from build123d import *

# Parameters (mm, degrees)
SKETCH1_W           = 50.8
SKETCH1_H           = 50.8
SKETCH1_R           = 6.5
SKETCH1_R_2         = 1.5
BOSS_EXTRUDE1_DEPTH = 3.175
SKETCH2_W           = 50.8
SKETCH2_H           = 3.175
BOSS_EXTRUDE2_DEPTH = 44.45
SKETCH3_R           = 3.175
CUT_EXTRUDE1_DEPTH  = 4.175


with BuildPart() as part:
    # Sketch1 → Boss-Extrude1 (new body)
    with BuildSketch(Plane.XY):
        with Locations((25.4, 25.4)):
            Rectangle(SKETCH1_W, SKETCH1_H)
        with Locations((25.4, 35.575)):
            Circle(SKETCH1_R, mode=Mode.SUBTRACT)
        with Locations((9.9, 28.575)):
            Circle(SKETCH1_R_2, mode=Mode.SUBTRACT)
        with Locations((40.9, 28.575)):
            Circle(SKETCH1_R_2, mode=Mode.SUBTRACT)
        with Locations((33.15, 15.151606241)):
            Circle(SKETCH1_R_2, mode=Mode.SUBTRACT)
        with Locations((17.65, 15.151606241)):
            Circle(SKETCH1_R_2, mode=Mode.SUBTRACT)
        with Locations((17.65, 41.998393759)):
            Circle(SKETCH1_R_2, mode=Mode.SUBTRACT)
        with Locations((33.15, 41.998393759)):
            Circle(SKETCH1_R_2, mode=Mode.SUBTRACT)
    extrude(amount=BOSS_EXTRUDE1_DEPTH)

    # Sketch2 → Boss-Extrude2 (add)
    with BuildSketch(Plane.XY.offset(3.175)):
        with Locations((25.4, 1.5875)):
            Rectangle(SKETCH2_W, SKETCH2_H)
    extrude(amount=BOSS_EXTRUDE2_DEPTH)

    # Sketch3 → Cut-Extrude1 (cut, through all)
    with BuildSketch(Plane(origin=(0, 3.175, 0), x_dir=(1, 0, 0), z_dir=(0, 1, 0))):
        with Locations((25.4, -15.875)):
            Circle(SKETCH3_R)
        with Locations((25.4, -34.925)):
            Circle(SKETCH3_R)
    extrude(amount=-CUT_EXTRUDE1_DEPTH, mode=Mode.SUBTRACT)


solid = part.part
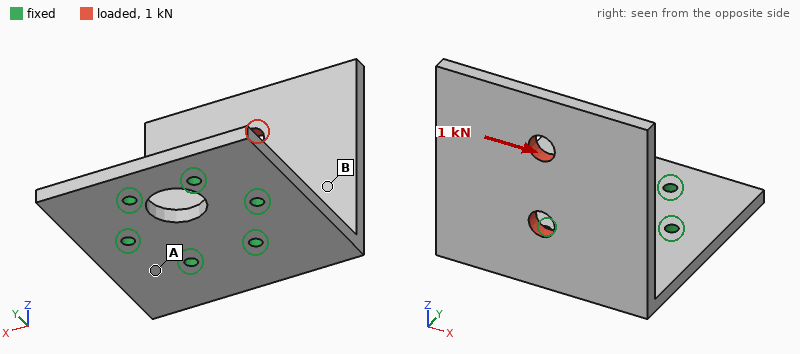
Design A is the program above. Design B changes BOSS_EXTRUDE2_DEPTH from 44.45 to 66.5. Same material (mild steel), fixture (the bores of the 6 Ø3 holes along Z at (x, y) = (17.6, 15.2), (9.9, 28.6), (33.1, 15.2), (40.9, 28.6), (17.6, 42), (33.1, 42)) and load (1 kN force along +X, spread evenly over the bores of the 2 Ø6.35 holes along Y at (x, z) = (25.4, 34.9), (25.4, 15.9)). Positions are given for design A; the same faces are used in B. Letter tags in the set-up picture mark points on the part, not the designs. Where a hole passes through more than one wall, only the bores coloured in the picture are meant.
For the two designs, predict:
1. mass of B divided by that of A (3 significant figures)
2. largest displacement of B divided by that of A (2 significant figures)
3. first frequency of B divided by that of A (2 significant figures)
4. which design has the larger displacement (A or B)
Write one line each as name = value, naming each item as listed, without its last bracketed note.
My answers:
mass of B divided by that of A = 1.24
largest displacement of B divided by that of A = 1.3
first frequency of B divided by that of A = 0.50
which design has the larger displacement = B
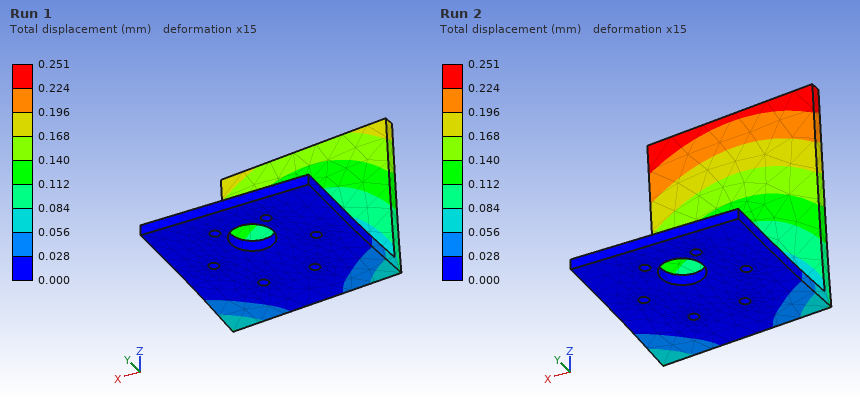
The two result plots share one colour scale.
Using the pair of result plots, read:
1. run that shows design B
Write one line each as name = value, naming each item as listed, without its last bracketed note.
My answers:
run that shows design B = Run 2
